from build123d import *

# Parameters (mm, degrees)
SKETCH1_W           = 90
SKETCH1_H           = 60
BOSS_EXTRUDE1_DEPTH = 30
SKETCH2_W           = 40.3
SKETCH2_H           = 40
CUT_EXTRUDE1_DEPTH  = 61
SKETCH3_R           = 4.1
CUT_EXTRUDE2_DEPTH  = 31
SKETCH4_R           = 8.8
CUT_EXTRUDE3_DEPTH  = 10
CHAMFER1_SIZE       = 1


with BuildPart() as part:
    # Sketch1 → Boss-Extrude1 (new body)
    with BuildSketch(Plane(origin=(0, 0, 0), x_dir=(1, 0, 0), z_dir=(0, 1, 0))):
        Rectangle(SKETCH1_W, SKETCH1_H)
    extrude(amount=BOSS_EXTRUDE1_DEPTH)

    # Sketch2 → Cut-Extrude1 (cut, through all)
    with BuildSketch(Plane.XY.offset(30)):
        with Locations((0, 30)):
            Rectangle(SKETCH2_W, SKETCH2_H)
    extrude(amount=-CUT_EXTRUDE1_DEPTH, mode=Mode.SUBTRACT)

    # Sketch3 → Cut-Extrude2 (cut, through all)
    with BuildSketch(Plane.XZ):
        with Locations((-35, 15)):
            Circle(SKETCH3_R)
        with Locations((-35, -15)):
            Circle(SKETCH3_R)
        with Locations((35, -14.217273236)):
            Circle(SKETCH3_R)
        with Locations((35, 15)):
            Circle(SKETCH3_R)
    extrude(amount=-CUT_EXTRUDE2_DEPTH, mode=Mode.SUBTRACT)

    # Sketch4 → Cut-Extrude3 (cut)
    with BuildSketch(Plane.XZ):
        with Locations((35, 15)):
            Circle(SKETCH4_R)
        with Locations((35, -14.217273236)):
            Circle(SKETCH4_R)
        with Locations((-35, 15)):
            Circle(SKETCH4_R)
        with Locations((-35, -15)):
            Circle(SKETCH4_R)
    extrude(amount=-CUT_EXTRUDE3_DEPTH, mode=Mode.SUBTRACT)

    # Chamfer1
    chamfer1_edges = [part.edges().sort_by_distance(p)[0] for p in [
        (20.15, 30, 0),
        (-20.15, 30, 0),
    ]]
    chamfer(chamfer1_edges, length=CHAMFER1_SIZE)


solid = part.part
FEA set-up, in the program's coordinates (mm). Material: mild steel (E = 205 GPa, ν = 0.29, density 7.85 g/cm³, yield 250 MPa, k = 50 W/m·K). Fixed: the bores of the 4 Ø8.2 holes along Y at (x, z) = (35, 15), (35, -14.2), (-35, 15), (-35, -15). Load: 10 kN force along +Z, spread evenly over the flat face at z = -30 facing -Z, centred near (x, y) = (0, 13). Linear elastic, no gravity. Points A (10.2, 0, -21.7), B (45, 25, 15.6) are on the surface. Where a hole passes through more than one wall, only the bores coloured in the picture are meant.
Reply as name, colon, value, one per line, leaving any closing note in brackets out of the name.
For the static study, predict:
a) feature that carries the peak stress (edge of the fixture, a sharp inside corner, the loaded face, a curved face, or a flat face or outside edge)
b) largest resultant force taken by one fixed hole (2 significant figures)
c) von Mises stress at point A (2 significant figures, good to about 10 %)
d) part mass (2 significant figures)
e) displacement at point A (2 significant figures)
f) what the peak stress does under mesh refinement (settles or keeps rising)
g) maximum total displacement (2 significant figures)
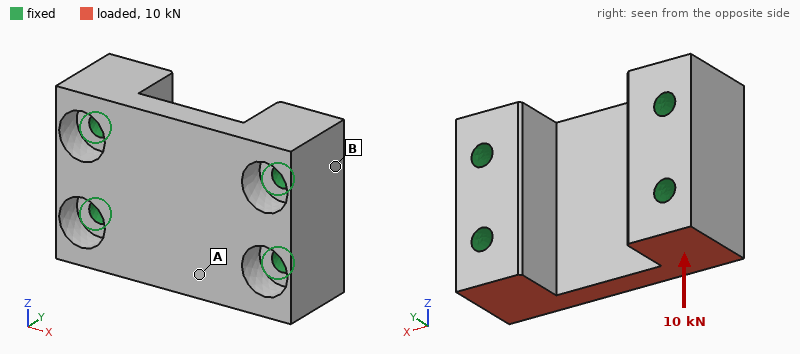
feature that carries the peak stress: edge of the fixture
largest resultant force taken by one fixed hole: 3.9 kN
von Mises stress at point A: 5.1 MPa
part mass: 780 g
displacement at point A: 1.7 µm
what the peak stress does under mesh refinement: keeps rising
maximum total displacement: 2.4 µm
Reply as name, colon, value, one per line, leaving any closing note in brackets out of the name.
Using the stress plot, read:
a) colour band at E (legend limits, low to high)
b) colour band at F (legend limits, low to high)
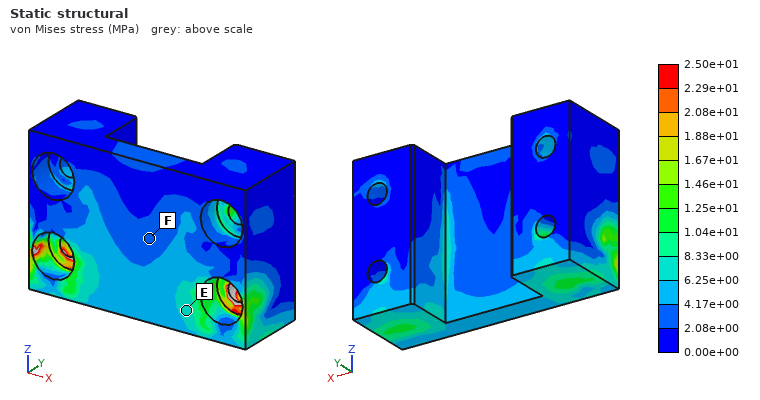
colour band at E: 6.25e+00 to 8.33e+00 MPa
colour band at F: 2.08e+00 to 4.17e+00 MPa
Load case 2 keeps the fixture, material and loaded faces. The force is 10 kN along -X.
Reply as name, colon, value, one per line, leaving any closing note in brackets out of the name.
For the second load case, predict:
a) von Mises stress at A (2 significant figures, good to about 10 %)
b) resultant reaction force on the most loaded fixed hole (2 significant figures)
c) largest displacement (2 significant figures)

von Mises stress at A: 8.7 MPa
resultant reaction force on the most loaded fixed hole: 5.0 kN
largest displacement: 4.0 µm
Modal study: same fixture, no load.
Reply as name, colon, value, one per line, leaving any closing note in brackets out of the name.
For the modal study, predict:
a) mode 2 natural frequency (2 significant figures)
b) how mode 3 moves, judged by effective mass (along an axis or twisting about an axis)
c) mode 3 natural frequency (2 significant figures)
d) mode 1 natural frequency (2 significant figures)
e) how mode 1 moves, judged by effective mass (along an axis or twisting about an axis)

mode 2 natural frequency: 16 kHz
how mode 3 moves, judged by effective mass: along X
mode 3 natural frequency: 19 kHz
mode 1 natural frequency: 15 kHz
how mode 1 moves, judged by effective mass: along Y
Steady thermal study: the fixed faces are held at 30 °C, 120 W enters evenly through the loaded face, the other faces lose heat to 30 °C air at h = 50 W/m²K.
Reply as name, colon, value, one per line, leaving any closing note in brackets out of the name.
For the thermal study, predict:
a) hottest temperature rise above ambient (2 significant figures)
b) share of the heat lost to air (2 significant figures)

hottest temperature rise above ambient: 37 K
share of the heat lost to air: 6.5 %
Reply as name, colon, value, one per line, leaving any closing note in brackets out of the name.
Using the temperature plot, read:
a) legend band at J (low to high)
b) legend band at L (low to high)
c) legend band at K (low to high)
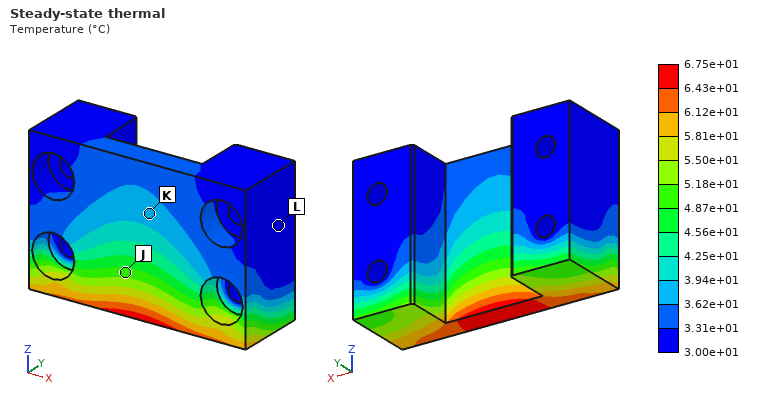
legend band at J: 4.87e+01 to 5.18e+01 °C
legend band at L: 3.00e+01 to 3.31e+01 °C
legend band at K: 3.62e+01 to 3.94e+01 °C
